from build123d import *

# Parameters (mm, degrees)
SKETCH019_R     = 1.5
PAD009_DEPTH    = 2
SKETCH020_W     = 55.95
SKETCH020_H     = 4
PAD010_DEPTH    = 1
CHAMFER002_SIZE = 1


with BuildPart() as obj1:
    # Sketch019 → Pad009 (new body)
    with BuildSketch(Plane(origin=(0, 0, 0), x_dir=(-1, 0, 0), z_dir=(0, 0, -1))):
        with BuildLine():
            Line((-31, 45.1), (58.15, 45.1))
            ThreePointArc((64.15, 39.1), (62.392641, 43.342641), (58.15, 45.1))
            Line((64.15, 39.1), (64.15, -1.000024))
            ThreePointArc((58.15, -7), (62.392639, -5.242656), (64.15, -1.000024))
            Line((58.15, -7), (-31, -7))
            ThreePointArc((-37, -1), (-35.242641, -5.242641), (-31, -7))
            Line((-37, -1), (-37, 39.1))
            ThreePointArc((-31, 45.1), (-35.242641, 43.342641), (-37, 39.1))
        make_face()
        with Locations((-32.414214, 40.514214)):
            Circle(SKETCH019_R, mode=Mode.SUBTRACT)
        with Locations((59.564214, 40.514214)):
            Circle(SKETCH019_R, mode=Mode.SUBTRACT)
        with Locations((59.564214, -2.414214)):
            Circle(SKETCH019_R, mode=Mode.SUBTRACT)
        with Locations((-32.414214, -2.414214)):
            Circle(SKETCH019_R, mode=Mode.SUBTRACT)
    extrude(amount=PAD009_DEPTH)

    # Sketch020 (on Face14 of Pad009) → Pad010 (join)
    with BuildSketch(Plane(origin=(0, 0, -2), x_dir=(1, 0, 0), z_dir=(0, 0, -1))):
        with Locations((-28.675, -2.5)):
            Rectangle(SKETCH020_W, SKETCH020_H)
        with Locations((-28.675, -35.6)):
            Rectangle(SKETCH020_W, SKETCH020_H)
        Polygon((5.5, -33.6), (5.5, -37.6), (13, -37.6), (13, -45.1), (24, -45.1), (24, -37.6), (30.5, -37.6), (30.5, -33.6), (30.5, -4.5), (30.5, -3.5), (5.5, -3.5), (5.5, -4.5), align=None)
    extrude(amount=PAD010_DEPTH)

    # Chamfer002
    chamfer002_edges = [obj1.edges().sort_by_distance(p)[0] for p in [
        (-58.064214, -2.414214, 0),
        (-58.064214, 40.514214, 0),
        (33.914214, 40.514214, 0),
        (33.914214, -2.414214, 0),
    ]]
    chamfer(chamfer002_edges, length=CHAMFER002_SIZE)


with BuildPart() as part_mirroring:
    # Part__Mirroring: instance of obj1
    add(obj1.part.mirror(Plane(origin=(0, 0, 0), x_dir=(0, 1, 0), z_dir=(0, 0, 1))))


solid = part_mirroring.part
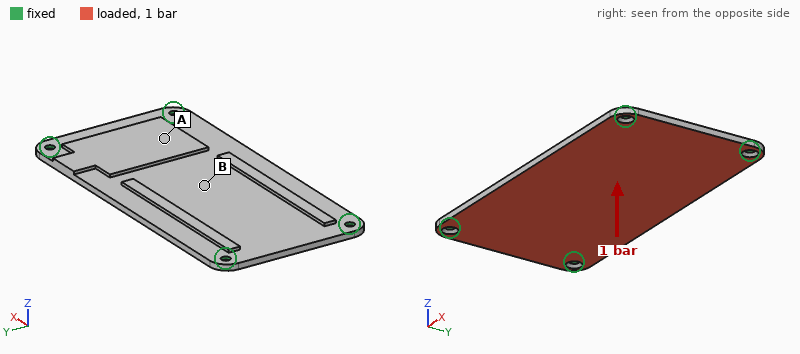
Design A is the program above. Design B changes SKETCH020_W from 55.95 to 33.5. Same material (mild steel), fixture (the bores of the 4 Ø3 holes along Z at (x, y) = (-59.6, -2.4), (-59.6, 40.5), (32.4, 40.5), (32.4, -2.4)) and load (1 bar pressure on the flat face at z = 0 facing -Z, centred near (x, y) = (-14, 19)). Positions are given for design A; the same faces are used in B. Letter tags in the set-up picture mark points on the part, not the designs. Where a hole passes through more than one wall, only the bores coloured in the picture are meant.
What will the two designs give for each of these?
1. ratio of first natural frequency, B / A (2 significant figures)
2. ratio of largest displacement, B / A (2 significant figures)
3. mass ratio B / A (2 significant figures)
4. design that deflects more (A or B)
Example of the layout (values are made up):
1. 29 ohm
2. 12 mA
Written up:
1. 0.97
2. 1.1
3. 0.98
4. B
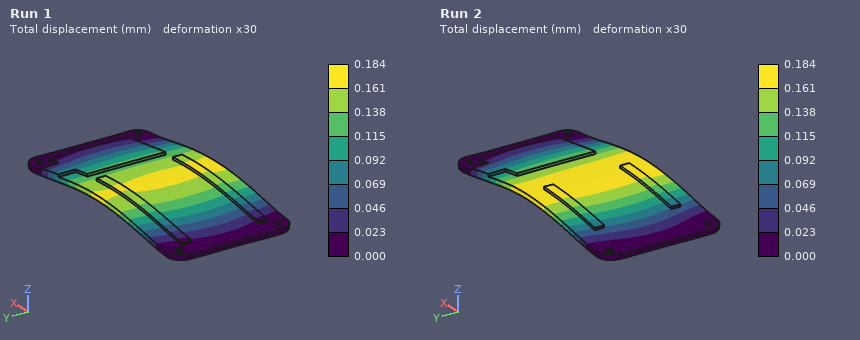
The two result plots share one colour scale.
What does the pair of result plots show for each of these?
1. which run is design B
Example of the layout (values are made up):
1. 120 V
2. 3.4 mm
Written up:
1. Run 2
